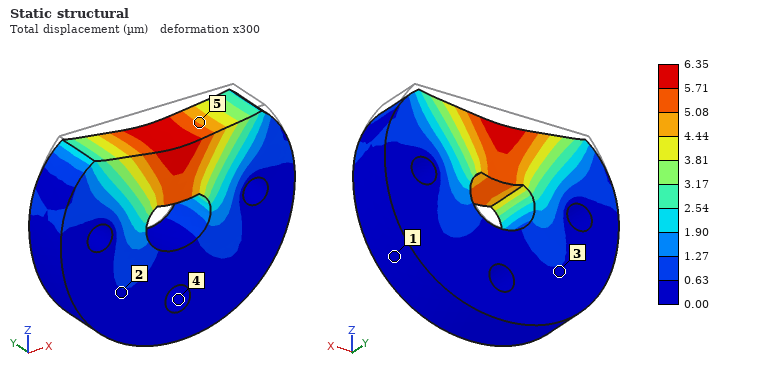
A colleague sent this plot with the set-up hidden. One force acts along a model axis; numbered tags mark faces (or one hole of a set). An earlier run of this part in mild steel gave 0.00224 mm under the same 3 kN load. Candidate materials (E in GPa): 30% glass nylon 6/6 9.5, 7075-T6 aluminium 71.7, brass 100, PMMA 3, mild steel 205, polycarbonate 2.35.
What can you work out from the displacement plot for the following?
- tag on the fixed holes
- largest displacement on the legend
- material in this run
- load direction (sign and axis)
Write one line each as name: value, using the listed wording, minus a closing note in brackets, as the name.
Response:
tag on the fixed holes: 4
largest displacement on the legend: 6.35 µm
material in this run: 7075-T6 aluminium
load direction: -Z
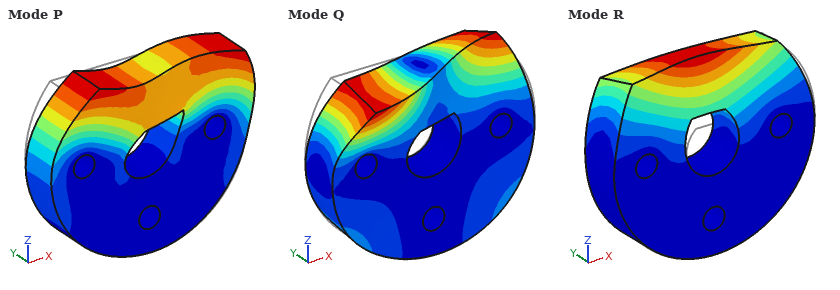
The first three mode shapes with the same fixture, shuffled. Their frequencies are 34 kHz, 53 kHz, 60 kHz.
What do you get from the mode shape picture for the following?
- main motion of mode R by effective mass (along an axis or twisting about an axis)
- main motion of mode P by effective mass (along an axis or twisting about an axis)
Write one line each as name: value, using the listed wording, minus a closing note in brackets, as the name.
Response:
main motion of mode R by effective mass: along Y
main motion of mode P by effective mass: along X
